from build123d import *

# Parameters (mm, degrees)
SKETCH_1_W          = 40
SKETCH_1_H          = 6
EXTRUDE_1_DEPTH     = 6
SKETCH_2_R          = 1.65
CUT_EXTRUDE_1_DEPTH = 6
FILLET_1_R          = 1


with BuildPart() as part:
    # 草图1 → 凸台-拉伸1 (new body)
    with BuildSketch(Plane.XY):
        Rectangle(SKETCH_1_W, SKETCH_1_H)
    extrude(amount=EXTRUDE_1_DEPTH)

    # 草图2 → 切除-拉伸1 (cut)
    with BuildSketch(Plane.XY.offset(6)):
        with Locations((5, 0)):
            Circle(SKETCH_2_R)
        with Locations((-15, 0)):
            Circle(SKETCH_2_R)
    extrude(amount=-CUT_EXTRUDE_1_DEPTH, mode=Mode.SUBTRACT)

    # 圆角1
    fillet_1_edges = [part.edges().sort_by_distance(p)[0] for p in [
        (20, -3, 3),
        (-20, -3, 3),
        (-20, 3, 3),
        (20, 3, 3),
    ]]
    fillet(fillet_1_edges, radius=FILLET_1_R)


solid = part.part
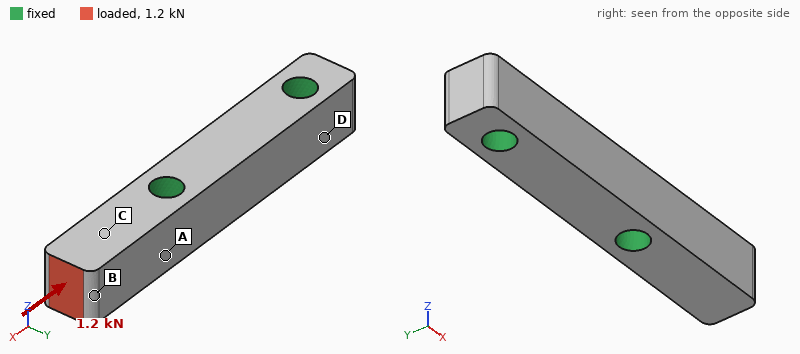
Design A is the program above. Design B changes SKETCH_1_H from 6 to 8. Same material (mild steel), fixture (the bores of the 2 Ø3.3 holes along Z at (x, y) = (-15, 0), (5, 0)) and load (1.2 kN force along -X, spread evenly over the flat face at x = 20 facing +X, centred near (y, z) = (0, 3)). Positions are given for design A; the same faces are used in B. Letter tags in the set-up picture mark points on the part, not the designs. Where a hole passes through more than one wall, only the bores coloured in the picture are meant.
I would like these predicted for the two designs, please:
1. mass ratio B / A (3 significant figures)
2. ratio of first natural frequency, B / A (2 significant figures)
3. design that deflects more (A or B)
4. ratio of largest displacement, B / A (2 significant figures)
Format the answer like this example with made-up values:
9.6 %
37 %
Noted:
1.36
1.1
A
0.77
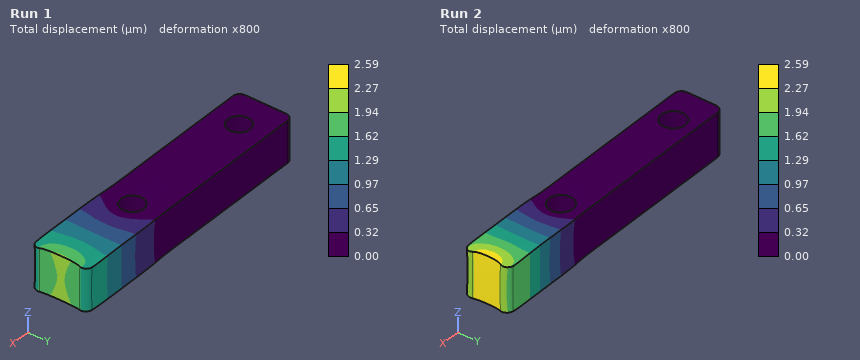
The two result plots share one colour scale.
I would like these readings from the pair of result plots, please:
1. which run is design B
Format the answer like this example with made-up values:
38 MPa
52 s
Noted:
Run 1
